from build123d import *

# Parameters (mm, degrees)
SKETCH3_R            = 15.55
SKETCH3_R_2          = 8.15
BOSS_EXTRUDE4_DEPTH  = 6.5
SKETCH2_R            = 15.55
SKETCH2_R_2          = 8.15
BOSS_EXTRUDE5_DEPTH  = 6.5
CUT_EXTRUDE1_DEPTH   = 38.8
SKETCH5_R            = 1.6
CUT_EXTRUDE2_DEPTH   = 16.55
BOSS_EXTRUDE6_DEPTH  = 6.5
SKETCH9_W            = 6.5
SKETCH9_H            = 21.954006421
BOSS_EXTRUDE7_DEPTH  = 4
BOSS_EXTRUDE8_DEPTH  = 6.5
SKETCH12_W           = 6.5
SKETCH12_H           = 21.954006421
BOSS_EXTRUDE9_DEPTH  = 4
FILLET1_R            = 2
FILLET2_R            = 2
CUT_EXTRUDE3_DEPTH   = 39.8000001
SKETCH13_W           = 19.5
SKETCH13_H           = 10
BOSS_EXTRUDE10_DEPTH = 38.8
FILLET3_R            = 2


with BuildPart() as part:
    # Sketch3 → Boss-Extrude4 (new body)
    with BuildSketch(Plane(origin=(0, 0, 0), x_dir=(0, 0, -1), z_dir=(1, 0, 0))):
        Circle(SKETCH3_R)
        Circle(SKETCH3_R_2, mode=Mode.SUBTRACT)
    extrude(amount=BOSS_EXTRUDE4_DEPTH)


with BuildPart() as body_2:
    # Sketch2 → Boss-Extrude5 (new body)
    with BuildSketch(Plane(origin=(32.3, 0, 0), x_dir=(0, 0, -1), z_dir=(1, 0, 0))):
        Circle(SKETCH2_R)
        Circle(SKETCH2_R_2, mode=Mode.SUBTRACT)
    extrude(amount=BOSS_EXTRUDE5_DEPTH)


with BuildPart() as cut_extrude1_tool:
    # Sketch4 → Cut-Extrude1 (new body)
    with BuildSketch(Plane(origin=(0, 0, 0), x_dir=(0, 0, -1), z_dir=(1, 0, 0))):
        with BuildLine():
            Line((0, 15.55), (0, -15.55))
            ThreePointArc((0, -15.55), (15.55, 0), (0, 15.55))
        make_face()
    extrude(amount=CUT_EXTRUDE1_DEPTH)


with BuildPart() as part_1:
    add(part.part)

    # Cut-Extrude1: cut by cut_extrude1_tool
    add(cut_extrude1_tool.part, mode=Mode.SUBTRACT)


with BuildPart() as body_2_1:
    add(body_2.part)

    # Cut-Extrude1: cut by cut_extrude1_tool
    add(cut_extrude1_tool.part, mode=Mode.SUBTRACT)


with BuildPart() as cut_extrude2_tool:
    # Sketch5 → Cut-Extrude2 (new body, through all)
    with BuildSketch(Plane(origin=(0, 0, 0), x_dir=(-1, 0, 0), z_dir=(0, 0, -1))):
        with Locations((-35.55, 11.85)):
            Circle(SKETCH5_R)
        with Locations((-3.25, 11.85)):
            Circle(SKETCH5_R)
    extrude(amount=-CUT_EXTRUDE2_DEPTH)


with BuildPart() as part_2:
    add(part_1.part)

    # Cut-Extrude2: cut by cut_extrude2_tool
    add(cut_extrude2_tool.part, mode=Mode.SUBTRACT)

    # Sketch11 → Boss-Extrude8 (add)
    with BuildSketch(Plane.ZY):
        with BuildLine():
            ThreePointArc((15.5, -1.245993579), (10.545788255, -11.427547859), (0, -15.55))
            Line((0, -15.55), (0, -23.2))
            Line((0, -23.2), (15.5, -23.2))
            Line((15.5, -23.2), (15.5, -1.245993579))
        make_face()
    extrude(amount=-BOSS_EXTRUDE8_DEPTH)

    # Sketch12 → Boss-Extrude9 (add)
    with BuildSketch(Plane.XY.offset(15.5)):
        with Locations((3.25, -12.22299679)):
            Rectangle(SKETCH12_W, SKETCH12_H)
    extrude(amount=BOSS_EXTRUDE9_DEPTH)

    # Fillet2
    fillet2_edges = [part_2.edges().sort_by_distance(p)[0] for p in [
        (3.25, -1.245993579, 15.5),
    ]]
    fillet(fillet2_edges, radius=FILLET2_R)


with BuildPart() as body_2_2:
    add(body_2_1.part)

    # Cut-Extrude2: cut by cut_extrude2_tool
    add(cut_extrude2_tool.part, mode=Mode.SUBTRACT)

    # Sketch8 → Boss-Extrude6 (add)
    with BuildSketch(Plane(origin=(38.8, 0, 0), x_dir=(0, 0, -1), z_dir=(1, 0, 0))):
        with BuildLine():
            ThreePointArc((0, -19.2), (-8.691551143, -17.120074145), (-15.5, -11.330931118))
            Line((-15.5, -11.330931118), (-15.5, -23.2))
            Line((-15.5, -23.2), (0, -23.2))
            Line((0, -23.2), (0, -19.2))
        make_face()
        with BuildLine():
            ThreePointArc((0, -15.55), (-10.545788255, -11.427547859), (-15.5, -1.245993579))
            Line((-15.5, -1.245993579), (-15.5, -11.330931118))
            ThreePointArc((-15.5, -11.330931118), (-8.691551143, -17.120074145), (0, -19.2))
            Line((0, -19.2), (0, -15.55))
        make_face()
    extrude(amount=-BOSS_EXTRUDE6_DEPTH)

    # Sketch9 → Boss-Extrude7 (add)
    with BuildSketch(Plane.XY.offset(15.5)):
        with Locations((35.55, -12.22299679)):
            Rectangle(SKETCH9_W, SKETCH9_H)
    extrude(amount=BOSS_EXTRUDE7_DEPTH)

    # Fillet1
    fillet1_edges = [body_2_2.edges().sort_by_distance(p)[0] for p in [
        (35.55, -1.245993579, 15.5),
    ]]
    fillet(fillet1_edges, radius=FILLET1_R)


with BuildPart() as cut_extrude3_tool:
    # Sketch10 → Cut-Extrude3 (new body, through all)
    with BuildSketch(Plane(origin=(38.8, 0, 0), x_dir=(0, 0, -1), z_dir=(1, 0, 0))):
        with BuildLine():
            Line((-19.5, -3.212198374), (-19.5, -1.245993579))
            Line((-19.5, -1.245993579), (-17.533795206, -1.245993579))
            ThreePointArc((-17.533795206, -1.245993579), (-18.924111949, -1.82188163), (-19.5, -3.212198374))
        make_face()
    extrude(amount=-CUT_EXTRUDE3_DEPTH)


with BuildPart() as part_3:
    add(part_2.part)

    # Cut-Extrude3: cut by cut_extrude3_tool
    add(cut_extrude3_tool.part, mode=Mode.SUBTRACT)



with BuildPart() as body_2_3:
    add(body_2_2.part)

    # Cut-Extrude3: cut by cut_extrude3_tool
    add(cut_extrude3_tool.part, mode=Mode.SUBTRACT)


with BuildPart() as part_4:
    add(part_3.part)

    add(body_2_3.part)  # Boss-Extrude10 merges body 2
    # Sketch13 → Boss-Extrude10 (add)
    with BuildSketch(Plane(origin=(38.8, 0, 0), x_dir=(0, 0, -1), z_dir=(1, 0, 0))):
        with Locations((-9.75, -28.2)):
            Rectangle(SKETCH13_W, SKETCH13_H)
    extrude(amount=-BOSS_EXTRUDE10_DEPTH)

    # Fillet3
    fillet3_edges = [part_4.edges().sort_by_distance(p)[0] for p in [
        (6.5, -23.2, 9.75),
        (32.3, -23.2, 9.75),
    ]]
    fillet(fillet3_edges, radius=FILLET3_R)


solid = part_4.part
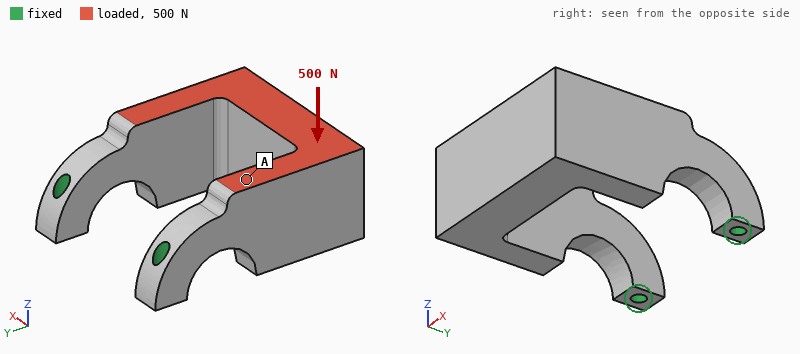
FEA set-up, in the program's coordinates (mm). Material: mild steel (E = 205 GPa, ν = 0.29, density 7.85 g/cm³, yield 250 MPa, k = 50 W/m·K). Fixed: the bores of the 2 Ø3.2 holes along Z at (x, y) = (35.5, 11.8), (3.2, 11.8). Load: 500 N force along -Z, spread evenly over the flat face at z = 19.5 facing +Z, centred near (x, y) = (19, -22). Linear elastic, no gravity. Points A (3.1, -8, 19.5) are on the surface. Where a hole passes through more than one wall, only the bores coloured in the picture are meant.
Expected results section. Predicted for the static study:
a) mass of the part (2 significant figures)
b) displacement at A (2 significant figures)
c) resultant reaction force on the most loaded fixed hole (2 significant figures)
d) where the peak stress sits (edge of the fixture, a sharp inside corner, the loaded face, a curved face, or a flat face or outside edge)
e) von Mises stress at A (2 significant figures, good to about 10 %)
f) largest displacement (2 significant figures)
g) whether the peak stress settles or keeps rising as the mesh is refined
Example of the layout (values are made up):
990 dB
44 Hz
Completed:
110 g
33 µm
250 N
edge of the fixture
15 MPa
84 µm
keeps rising
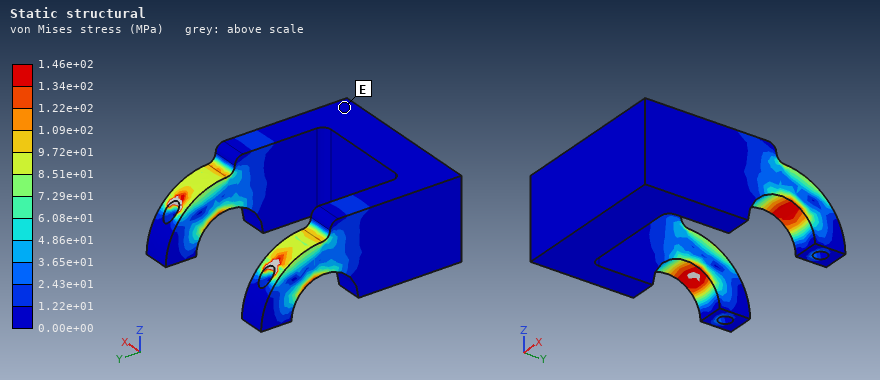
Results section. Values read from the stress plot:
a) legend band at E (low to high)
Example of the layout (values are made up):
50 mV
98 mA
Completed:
0.00e+00 to 1.22e+01 MPa
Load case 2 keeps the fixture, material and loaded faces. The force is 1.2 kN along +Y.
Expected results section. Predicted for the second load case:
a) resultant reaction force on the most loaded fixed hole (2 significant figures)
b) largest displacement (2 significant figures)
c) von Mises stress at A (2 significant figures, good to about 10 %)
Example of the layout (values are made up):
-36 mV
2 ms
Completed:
600 N
70 µm
20 MPa
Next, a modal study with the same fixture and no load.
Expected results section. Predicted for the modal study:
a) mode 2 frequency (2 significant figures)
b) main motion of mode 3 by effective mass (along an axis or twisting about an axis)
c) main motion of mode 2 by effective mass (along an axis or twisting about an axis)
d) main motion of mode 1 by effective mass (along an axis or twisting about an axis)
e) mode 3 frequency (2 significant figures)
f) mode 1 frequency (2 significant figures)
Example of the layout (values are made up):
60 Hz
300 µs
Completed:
2500 Hz
twisting about Y
along X
along Z
4600 Hz
1400 Hz
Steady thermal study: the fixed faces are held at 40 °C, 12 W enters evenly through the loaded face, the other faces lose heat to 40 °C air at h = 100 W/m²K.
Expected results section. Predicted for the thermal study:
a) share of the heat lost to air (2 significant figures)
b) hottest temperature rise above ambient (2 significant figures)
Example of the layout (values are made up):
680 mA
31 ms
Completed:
65 %
24 K
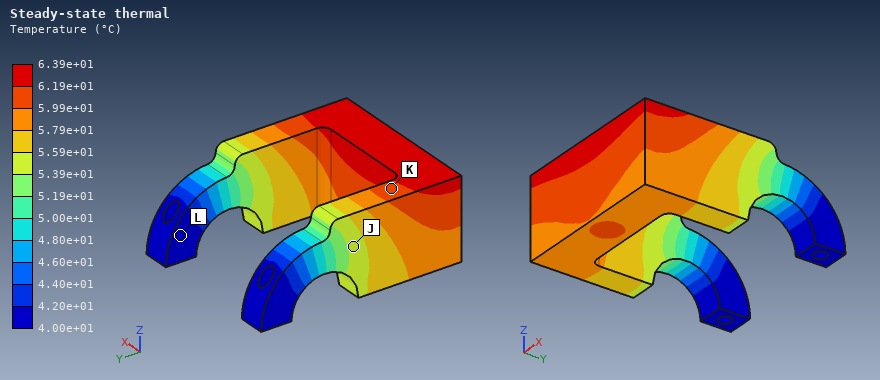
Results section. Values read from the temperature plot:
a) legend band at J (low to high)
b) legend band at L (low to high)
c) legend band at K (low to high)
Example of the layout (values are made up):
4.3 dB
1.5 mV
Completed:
5.39e+01 to 5.59e+01 °C
4.00e+01 to 4.20e+01 °C
5.99e+01 to 6.19e+01 °C
